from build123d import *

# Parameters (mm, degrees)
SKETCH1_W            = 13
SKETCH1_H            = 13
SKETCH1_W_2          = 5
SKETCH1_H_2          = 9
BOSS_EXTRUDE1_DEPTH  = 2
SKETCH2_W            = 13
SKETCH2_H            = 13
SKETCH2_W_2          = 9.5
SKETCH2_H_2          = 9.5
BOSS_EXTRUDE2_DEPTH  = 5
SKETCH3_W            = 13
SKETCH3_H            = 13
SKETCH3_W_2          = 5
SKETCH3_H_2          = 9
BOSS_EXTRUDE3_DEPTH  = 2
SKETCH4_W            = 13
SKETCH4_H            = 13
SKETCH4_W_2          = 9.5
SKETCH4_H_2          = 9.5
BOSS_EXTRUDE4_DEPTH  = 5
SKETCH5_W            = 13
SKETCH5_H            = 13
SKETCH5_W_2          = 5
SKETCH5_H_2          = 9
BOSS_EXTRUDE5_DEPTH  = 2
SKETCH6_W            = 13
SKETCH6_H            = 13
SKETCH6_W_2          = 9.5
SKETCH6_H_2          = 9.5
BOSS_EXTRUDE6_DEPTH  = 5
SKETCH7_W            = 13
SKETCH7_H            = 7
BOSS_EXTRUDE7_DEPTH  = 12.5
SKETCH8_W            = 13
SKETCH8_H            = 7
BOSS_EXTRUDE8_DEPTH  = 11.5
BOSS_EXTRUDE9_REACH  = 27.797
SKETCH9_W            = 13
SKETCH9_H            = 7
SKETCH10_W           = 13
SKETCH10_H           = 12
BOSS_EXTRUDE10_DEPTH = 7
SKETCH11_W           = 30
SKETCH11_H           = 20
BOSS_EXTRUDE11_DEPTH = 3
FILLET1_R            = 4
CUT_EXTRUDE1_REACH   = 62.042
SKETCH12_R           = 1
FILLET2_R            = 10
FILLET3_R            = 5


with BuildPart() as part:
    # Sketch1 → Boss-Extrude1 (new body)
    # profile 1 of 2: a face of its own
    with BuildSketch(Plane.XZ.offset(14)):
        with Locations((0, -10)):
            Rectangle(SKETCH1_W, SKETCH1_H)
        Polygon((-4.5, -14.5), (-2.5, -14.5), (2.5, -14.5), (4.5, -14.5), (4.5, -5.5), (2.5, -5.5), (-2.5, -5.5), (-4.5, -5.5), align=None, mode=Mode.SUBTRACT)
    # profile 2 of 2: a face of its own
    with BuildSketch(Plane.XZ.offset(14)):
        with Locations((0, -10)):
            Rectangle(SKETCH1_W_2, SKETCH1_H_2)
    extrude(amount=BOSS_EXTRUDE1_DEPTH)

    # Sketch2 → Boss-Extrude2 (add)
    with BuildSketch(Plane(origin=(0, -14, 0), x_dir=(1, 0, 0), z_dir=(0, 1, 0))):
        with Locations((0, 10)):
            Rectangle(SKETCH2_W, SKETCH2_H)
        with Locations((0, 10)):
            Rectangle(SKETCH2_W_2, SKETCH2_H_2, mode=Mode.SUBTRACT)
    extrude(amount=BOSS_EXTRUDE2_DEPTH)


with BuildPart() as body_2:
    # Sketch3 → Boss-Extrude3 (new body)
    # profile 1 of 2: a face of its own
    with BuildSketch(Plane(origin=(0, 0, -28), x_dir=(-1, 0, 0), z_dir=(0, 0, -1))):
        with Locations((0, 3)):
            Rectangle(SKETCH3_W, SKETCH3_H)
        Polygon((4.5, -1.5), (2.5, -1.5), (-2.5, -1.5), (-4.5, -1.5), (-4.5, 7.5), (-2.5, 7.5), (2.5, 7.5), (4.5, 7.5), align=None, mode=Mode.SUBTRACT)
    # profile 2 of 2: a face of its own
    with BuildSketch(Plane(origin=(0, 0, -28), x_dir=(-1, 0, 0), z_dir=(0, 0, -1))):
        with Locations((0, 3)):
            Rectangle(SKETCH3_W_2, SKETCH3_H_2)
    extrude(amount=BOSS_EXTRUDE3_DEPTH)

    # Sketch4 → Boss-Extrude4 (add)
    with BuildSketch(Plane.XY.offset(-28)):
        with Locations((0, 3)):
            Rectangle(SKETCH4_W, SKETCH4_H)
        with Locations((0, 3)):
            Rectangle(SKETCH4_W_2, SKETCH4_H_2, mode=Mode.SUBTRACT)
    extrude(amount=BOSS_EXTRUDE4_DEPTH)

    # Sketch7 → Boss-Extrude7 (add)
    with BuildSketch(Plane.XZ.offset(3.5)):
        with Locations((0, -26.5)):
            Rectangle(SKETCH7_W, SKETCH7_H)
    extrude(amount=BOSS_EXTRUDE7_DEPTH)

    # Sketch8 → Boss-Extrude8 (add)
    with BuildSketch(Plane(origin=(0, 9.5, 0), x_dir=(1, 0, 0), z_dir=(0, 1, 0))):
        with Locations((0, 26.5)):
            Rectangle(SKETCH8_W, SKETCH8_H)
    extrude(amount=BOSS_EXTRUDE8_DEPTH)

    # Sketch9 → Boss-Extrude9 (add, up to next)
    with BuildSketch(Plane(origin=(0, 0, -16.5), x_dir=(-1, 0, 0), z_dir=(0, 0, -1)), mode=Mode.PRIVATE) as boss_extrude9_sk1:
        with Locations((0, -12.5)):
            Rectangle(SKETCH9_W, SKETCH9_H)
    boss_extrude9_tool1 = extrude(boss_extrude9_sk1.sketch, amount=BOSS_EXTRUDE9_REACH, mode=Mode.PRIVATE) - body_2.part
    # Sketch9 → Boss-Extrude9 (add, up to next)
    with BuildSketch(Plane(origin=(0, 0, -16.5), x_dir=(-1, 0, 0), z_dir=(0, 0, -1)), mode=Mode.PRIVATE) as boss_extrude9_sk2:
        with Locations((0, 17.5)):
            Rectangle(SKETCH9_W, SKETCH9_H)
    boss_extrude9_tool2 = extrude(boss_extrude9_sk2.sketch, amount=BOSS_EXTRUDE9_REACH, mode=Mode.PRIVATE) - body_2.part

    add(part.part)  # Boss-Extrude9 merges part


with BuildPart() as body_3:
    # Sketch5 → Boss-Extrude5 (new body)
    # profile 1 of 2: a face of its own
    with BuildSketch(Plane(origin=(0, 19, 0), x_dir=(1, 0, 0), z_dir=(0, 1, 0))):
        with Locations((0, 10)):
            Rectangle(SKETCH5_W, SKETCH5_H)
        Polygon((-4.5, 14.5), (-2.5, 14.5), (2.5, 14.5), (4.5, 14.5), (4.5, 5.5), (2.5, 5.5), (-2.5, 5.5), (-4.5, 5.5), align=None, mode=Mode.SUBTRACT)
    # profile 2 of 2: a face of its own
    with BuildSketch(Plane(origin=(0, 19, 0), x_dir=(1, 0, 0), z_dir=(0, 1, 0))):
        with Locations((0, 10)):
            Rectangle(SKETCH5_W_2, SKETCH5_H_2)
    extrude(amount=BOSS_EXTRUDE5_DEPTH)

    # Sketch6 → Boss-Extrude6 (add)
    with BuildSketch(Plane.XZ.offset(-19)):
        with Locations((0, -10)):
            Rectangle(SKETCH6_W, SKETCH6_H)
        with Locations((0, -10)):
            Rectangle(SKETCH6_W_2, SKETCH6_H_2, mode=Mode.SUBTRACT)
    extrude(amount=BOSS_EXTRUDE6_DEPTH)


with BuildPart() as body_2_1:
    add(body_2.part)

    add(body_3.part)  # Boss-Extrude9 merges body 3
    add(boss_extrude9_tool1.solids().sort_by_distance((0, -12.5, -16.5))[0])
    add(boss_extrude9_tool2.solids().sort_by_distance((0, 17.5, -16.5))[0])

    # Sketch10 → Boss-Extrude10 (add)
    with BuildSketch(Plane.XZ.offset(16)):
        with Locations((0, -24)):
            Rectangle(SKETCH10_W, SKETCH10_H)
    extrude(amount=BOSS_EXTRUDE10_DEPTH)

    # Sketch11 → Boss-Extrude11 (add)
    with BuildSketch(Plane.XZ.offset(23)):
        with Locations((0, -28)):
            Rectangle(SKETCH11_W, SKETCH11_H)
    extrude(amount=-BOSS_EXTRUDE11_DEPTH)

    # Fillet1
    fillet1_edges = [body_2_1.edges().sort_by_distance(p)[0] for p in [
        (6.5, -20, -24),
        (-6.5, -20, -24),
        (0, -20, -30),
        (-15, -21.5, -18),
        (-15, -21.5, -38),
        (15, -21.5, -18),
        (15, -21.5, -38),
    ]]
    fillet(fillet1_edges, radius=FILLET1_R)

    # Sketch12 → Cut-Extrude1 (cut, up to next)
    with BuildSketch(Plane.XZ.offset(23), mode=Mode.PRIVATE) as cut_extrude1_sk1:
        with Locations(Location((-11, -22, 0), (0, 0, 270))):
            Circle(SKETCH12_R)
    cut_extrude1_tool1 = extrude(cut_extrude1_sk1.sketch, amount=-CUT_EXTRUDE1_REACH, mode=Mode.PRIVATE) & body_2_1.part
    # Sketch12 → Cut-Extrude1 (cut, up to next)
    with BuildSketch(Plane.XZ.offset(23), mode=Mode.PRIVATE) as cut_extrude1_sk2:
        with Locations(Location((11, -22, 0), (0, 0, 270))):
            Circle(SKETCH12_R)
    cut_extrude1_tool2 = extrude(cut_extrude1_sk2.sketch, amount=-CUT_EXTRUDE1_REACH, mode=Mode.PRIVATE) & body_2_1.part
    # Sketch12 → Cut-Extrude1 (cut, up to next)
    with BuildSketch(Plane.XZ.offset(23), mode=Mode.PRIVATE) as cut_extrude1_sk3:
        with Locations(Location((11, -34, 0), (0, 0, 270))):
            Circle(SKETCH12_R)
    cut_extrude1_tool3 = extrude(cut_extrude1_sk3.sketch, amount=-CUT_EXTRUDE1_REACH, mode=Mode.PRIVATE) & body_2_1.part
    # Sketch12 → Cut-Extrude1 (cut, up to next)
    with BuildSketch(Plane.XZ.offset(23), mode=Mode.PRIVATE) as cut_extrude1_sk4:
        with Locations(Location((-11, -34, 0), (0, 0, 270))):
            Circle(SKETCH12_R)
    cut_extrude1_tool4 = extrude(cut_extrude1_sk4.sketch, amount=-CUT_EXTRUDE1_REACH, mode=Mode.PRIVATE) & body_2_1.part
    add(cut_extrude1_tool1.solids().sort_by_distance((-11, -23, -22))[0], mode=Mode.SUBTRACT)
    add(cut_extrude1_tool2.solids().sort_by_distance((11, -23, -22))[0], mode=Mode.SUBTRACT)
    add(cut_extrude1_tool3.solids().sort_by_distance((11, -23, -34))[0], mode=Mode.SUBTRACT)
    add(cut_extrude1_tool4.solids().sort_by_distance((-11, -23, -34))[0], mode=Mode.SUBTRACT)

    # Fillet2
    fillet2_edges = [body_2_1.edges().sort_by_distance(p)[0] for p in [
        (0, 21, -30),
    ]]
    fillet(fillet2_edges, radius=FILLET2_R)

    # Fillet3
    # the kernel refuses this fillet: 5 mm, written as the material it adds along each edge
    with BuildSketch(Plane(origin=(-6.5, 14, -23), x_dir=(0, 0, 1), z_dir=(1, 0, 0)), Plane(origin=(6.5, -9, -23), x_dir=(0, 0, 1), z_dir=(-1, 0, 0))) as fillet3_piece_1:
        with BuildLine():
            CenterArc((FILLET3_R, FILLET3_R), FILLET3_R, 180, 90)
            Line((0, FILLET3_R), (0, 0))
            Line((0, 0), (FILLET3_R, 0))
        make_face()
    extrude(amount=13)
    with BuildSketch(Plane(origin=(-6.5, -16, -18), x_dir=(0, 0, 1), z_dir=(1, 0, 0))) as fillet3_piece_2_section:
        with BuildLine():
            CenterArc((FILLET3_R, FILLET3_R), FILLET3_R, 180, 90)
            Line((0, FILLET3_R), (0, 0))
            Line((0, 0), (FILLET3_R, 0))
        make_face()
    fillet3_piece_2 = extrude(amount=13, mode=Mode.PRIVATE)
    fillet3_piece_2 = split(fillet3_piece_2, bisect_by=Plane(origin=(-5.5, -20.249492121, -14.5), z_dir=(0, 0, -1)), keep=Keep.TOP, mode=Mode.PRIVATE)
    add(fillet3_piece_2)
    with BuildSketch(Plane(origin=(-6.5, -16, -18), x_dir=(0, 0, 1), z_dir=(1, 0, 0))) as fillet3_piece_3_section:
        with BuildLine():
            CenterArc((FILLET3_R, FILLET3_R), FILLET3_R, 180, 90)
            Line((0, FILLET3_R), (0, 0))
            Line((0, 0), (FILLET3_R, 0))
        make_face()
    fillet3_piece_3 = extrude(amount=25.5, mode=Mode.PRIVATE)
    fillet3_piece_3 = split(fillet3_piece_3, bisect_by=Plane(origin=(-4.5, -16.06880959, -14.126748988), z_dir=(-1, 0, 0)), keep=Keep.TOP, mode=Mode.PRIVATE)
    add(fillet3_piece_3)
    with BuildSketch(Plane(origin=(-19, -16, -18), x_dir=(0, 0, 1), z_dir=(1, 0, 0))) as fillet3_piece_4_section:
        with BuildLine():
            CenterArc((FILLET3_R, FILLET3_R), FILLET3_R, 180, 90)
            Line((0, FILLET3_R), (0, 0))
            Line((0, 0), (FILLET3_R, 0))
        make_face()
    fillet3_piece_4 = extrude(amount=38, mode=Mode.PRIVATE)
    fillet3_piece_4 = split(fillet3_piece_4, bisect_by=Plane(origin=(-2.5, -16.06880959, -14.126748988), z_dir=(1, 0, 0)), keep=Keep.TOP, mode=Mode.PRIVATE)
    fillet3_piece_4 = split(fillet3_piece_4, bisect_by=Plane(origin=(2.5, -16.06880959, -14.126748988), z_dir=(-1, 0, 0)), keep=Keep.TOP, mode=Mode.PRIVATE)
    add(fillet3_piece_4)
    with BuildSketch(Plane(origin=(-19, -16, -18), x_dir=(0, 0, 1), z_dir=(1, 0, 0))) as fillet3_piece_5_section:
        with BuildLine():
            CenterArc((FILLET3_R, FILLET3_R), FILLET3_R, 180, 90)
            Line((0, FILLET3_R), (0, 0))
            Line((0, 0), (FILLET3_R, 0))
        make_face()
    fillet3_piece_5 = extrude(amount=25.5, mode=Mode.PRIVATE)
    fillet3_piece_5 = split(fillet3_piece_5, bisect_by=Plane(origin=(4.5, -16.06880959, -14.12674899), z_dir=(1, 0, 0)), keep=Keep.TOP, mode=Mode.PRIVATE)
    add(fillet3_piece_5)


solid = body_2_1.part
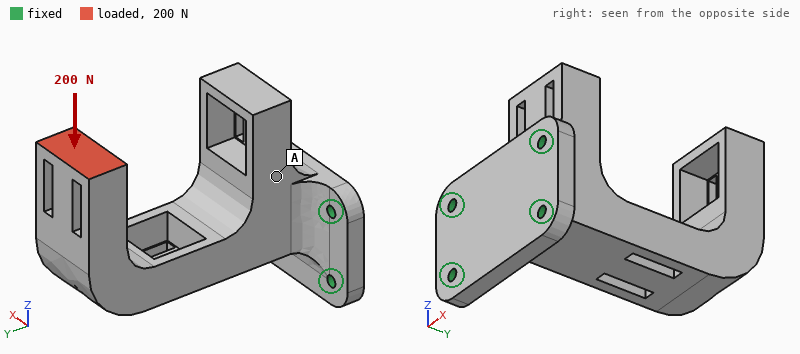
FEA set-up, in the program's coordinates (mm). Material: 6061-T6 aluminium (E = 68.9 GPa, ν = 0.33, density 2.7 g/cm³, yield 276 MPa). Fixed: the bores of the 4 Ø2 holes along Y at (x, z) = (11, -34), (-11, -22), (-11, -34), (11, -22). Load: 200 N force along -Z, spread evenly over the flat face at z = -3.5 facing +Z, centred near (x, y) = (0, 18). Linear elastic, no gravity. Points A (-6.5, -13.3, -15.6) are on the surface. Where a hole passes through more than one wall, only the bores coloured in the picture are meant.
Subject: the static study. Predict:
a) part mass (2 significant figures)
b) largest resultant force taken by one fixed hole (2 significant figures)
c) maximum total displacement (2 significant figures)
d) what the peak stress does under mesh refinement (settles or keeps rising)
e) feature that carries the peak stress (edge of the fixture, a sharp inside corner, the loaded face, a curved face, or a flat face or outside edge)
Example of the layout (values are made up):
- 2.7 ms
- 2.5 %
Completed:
- 21 g
- 340 N
- 0.23 mm
- keeps rising
- edge of the fixture
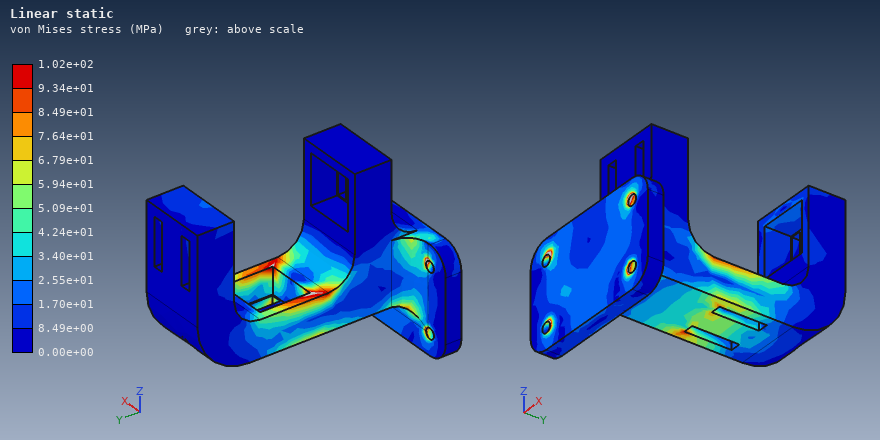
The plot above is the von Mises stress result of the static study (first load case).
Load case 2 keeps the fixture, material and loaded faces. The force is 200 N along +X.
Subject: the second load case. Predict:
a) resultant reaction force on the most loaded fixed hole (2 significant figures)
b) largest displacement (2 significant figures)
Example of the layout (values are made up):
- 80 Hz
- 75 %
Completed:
- 320 N
- 0.37 mm
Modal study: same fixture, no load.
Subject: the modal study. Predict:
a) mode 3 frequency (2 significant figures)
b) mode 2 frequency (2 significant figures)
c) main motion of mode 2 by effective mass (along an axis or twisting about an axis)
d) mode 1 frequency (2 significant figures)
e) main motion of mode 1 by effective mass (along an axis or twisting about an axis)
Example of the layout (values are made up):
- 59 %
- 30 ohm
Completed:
- 6700 Hz
- 2700 Hz
- along X
- 2200 Hz
- along Z
